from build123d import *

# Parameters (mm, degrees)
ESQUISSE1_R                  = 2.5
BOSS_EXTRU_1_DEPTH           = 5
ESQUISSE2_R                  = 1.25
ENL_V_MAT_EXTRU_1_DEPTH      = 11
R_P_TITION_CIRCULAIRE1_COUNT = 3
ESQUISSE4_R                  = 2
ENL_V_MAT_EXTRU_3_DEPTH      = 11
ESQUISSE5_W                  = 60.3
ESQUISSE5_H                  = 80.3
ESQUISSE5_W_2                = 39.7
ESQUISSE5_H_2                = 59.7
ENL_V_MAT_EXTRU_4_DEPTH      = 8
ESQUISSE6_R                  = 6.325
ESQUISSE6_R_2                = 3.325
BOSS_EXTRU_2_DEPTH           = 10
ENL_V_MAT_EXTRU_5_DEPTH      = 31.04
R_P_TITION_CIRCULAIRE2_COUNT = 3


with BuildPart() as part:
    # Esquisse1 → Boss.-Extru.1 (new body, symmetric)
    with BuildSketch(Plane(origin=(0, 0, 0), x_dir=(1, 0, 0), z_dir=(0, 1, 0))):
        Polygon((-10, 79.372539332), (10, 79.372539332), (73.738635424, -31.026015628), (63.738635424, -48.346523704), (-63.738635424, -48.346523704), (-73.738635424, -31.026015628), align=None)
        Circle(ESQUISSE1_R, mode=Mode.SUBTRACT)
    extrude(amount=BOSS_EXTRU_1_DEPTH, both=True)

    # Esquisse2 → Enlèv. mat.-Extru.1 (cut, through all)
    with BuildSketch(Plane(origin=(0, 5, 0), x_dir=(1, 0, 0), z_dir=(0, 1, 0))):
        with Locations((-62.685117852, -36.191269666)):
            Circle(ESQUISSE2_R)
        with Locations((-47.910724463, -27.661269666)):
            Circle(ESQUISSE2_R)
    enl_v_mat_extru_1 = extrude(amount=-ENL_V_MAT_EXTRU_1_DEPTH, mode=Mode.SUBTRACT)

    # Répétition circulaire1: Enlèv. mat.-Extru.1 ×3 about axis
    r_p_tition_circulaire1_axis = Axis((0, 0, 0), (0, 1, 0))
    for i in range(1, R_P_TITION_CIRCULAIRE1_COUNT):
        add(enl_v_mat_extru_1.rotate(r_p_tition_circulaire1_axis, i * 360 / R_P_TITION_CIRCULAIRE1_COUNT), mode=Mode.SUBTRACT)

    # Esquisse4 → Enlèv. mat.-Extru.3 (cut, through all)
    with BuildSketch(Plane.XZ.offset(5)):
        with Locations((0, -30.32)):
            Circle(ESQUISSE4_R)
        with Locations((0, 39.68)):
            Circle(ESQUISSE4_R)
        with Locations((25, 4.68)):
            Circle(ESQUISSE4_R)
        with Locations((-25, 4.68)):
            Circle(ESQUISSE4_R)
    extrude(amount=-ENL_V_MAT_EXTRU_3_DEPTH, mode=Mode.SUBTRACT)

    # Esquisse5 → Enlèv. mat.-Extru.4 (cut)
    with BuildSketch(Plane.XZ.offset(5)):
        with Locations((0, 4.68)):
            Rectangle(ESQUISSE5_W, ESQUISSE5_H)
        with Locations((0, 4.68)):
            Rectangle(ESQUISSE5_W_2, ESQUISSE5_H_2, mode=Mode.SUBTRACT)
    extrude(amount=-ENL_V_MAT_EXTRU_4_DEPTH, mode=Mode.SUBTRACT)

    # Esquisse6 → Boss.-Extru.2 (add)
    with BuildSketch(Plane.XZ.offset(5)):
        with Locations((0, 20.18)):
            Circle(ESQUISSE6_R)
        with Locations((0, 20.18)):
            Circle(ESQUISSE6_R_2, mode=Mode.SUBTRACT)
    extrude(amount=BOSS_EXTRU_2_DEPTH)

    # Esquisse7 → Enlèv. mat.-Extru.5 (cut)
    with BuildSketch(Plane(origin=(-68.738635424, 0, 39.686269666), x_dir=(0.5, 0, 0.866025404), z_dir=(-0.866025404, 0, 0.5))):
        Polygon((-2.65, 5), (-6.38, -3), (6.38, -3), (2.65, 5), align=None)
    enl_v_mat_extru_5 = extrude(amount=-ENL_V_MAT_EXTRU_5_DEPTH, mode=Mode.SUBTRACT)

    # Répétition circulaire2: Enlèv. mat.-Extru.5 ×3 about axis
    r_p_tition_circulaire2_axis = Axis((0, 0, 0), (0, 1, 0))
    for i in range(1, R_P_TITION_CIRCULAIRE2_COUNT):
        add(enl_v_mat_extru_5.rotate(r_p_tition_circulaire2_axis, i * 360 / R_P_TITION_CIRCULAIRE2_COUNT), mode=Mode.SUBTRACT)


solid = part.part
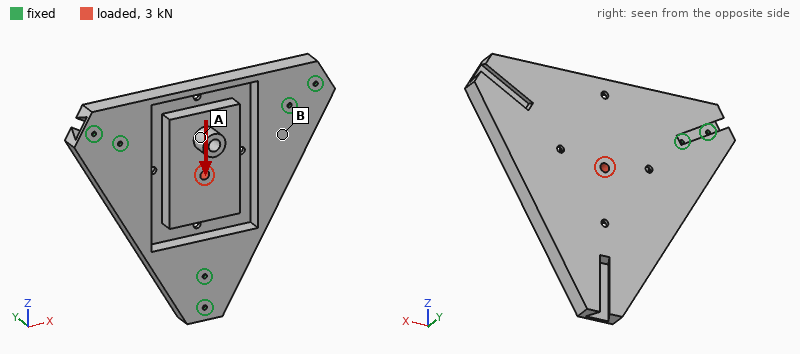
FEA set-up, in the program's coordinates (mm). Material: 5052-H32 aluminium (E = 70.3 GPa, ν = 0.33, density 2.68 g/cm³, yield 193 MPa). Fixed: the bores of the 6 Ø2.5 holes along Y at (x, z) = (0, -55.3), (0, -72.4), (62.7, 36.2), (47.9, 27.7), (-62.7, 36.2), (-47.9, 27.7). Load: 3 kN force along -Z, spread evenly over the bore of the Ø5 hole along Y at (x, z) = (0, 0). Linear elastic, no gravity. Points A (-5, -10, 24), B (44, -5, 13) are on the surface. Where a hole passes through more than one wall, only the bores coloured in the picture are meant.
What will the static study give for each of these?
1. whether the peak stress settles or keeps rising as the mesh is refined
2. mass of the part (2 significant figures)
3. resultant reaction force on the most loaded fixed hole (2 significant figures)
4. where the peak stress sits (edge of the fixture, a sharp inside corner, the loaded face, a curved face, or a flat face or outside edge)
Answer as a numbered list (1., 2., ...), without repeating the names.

1. keeps rising
2. 240 g
3. 830 N
4. edge of the fixture
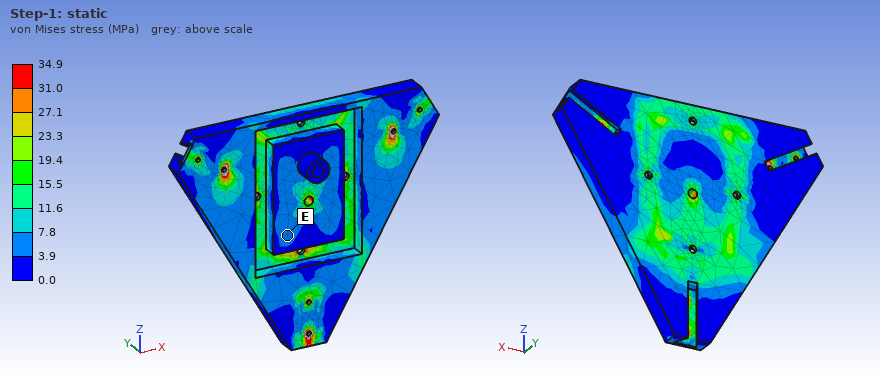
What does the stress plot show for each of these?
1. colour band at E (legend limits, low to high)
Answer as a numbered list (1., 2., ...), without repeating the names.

1. 3.9 to 7.8 MPa
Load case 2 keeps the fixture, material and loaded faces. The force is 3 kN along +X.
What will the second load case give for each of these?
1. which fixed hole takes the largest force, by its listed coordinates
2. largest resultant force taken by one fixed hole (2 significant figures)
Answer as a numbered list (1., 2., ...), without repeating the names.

1. (0, -55.3)
2. 860 N
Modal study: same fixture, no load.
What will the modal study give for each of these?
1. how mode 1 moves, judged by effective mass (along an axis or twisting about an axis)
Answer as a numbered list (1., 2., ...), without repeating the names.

1. along Y
